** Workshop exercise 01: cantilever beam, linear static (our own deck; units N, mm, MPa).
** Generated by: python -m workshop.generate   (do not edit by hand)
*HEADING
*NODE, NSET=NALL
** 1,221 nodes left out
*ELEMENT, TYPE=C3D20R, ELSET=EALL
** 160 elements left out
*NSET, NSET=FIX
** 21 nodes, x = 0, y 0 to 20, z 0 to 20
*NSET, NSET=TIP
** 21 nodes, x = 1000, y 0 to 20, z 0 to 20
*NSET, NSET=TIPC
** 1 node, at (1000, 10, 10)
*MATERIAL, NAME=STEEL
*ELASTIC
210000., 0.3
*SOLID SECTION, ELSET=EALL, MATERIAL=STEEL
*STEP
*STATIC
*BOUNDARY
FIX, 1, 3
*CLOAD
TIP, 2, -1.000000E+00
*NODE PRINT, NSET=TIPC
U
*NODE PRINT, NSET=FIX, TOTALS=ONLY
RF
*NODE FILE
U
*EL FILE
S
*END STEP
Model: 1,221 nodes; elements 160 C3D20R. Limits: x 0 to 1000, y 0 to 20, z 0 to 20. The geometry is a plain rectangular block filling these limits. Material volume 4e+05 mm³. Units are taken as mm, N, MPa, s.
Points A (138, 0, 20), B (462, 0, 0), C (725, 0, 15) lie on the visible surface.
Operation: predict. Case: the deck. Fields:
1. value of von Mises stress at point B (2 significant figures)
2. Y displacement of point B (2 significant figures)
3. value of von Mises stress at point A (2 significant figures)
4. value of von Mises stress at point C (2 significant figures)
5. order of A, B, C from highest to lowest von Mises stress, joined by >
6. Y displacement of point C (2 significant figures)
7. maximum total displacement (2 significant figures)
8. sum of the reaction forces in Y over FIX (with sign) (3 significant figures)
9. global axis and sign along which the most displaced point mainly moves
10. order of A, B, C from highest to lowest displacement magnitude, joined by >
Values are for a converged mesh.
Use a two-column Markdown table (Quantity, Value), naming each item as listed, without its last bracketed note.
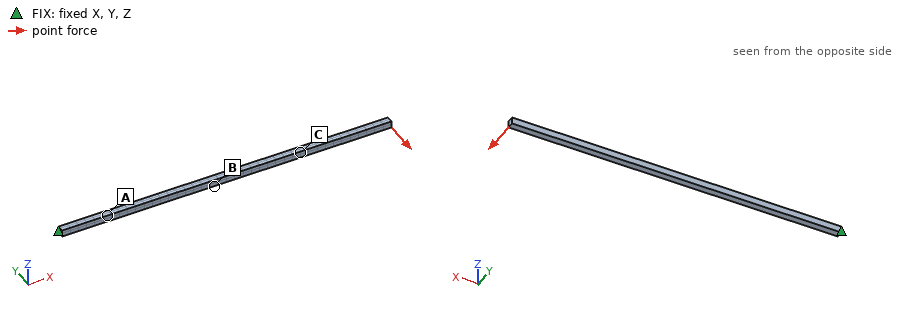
| Quantity | Value |
|---|---|
| value of von Mises stress at point B | 8.5 MPa |
| Y displacement of point B | -0.68 mm |
| value of von Mises stress at point A | 14 MPa |
| value of von Mises stress at point C | 4.3 MPa |
| order of A, B, C from highest to lowest von Mises stress, joined by > | A > B > C |
| Y displacement of point C | -1.5 mm |
| maximum total displacement | 2.5 mm |
| sum of the reaction forces in Y over FIX (with sign) | 21.0 N |
| global axis and sign along which the most displaced point mainly moves | -Y |
| order of A, B, C from highest to lowest displacement magnitude, joined by > | C > B > A |
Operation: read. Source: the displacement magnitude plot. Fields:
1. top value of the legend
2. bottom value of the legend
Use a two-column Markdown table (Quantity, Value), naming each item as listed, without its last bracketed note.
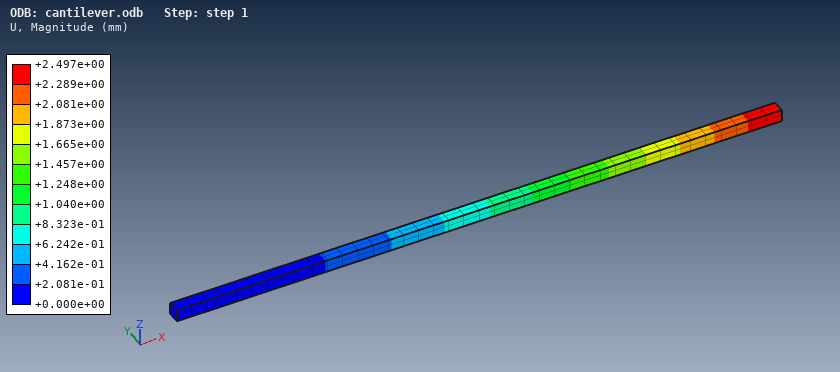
| Quantity | Value |
|---|---|
| top value of the legend | +2.497e+00 mm |
| bottom value of the legend | +0.000e+00 mm |
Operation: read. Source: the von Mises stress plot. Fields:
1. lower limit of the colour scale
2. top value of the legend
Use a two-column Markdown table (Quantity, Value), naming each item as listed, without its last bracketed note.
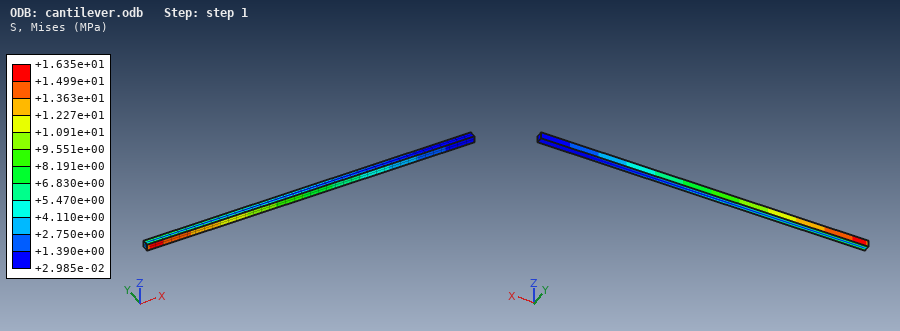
| Quantity | Value |
|---|---|
| lower limit of the colour scale | +2.985e-02 MPa |
| top value of the legend | +1.635e+01 MPa |
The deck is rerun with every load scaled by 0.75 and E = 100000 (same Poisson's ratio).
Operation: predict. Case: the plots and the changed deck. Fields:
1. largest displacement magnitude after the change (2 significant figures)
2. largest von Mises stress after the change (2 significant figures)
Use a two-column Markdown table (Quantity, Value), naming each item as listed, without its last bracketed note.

| Quantity | Value |
|---|---|
| largest displacement magnitude after the change | 3.9 mm |
| largest von Mises stress after the change | 12 MPa |
